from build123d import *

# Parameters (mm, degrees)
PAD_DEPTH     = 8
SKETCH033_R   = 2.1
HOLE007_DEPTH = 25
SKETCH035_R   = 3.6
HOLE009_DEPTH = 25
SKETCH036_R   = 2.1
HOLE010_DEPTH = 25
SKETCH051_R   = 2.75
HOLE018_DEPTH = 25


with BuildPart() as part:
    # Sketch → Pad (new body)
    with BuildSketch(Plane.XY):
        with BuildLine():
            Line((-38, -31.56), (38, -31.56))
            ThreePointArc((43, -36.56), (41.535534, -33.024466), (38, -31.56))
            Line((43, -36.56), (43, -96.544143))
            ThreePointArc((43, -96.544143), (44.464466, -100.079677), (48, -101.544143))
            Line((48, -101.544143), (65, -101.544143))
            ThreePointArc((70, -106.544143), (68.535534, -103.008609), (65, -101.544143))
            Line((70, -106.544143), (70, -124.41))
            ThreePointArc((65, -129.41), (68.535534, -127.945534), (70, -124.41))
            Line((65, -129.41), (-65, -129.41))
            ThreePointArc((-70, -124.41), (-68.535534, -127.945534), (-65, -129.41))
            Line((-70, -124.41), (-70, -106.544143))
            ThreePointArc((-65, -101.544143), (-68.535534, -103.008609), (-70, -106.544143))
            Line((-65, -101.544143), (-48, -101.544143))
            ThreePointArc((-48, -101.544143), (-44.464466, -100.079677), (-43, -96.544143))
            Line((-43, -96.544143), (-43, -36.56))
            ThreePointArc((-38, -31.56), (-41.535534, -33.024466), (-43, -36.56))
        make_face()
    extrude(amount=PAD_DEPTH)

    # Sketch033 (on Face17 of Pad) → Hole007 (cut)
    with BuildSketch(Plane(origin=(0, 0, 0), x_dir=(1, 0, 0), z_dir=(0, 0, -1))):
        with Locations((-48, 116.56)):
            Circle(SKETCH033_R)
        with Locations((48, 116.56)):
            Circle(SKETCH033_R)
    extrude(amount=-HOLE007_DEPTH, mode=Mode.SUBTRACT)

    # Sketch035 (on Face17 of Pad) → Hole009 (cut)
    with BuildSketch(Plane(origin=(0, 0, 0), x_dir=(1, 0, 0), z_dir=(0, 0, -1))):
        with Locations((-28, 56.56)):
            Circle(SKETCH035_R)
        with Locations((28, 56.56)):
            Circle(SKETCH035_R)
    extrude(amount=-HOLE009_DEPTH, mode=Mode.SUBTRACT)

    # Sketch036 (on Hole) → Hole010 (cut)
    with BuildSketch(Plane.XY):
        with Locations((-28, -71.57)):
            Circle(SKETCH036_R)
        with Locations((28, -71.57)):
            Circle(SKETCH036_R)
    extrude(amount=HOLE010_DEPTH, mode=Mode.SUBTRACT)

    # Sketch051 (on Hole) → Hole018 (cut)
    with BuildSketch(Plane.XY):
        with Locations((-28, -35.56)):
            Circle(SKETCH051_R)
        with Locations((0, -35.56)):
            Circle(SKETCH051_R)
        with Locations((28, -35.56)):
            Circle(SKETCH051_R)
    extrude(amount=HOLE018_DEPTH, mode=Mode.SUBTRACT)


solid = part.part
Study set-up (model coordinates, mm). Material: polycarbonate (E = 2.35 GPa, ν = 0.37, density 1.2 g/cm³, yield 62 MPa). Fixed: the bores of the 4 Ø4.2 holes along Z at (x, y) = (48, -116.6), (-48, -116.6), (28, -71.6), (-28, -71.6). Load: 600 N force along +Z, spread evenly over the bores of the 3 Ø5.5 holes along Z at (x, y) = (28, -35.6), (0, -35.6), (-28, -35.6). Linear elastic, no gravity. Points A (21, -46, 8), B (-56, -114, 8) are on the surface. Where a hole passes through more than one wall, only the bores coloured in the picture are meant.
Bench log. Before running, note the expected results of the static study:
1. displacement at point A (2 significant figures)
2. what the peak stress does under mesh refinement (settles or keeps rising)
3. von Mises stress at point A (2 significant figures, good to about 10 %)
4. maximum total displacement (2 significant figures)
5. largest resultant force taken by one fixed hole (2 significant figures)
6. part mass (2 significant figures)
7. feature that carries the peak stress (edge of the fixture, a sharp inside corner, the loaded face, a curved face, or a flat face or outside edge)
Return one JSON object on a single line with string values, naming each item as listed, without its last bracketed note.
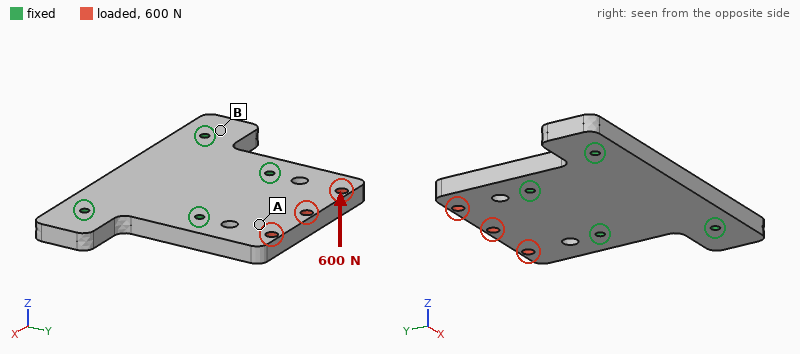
{"displacement at point A": "1.0 mm", "what the peak stress does under mesh refinement": "keeps rising", "von Mises stress at point A": "6.5 MPa", "maximum total displacement": "2.0 mm", "largest resultant force taken by one fixed hole": "390 N", "part mass": "93 g", "feature that carries the peak stress": "edge of the fixture"}
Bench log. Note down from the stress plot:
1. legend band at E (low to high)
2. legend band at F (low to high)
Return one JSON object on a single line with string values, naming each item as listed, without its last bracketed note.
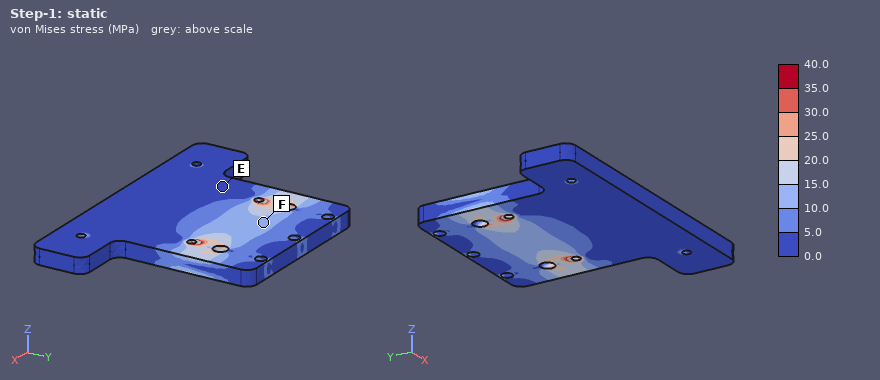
{"legend band at E": "0.0 to 5.0 MPa", "legend band at F": "10.0 to 15.0 MPa"}
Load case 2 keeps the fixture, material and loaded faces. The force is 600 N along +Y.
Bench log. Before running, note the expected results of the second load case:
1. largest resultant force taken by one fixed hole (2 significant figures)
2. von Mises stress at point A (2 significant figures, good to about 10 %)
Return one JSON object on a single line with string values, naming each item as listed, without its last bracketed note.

{"largest resultant force taken by one fixed hole": "260 N", "von Mises stress at point A": "1.2 MPa"}
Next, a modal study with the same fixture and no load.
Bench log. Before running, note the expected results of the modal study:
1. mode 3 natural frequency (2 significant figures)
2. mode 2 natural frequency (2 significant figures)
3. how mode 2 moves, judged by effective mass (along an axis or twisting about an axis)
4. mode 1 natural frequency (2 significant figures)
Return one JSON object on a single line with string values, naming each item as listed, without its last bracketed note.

{"mode 3 natural frequency": "1500 Hz", "mode 2 natural frequency": "1300 Hz", "how mode 2 moves, judged by effective mass": "along Z", "mode 1 natural frequency": "920 Hz"}
